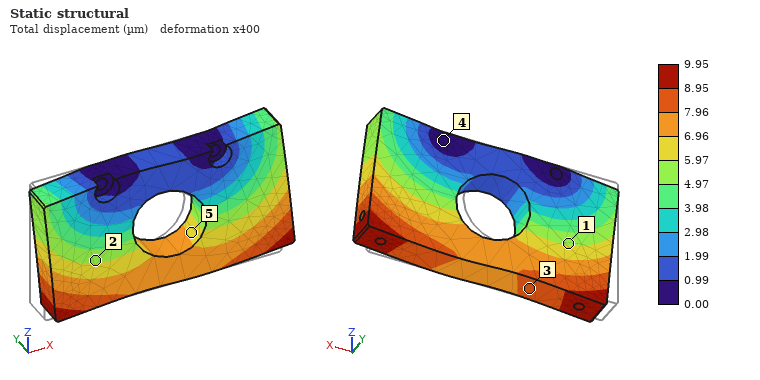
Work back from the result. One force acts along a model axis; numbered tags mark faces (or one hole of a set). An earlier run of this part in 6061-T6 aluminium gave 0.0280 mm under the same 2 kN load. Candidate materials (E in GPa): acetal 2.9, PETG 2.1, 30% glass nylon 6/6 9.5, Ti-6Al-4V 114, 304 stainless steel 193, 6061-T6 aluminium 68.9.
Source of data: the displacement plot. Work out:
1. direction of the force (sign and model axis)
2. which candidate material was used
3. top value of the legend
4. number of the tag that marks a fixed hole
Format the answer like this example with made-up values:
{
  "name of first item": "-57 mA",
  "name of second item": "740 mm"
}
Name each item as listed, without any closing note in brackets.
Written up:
{
  "direction of the force": "+X",
  "which candidate material was used": "304 stainless steel",
  "top value of the legend": "9.95 µm",
  "number of the tag that marks a fixed hole": "4"
}
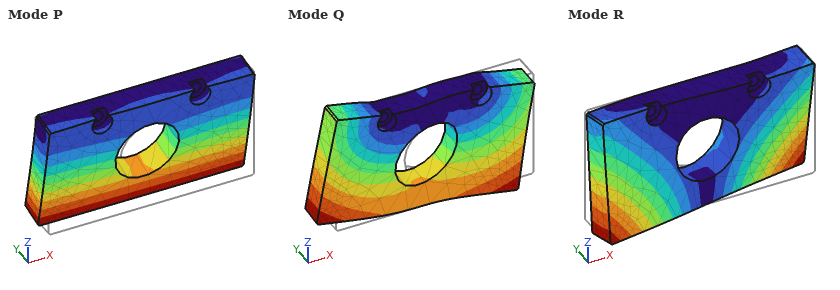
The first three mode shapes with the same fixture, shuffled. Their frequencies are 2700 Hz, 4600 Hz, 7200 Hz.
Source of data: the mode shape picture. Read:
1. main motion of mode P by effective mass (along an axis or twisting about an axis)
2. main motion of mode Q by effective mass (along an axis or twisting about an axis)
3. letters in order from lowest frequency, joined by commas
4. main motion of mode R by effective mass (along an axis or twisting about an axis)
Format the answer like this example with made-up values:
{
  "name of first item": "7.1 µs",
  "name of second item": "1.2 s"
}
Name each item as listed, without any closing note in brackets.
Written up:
{
  "main motion of mode P by effective mass": "along Y",
  "main motion of mode Q by effective mass": "along X",
  "letters in order from lowest frequency, joined by commas": "P, R, Q",
  "main motion of mode R by effective mass": "twisting about Z"
}
